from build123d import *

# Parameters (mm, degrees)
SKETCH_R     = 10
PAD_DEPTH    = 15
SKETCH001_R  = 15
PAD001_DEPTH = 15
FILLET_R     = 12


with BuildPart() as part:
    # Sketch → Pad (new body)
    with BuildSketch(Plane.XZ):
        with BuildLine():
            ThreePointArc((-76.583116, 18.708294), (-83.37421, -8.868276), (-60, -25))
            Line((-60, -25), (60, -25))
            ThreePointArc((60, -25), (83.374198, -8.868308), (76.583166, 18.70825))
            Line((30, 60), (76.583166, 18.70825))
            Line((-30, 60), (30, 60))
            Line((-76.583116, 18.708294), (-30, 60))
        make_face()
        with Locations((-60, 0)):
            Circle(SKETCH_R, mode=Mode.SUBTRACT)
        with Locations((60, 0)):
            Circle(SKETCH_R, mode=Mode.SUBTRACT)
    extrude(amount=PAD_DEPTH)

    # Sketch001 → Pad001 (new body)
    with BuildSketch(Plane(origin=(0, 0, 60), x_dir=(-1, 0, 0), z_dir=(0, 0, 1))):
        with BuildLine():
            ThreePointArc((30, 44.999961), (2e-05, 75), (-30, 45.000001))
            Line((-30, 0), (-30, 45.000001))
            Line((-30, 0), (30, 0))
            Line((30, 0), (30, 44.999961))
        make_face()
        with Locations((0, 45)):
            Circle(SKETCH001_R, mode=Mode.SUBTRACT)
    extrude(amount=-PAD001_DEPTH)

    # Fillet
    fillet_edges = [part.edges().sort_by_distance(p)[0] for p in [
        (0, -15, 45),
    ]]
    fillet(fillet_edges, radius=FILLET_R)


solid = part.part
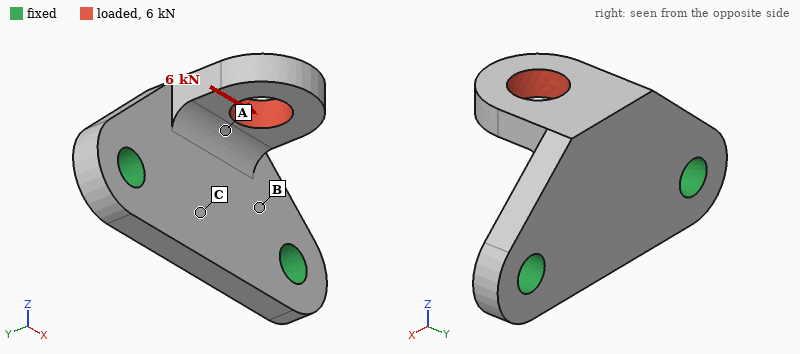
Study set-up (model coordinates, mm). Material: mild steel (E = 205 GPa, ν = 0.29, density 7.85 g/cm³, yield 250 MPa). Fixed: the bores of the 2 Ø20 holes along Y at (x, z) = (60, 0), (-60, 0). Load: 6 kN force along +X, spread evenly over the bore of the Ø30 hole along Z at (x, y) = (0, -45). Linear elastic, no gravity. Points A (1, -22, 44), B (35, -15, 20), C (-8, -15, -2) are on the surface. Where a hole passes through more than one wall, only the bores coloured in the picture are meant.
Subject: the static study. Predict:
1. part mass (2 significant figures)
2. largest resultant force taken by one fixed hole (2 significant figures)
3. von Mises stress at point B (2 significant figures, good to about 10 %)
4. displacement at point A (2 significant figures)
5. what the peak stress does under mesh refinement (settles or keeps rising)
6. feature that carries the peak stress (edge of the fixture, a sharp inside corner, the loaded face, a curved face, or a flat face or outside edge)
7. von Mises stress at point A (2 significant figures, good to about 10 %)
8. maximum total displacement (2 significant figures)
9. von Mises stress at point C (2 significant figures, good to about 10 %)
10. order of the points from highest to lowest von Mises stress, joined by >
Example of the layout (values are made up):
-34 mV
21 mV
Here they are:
1.6 kg
4.5 kN
20 MPa
9.7 µm
keeps rising
a sharp inside corner
45 MPa
48 µm
9.0 MPa
A > B > C
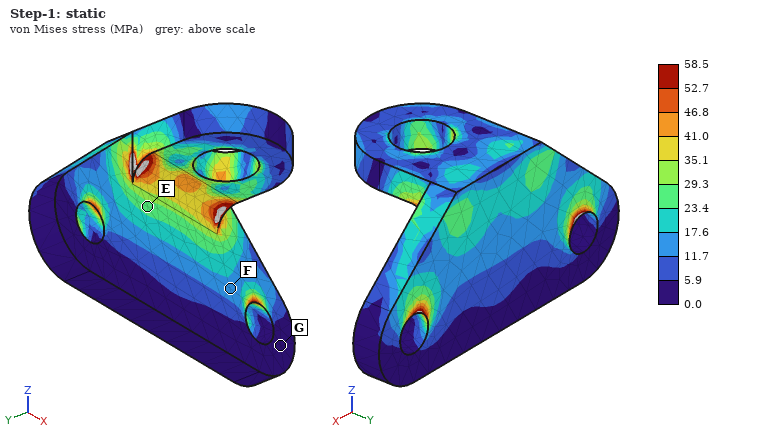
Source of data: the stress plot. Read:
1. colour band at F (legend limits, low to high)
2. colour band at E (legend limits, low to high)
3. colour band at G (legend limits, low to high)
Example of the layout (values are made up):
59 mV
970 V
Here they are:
11.7 to 17.6 MPa
23.4 to 29.3 MPa
0.0 to 5.9 MPa
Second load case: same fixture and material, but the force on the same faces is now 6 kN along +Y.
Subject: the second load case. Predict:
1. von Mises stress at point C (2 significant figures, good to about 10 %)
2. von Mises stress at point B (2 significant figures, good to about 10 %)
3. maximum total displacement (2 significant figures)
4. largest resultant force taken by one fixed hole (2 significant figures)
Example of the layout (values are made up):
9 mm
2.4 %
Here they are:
17 MPa
39 MPa
0.11 mm
3.0 kN
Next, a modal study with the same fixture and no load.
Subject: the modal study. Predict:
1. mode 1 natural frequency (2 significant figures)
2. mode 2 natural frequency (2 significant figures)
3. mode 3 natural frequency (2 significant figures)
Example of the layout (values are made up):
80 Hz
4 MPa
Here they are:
1800 Hz
3700 Hz
3700 Hz
